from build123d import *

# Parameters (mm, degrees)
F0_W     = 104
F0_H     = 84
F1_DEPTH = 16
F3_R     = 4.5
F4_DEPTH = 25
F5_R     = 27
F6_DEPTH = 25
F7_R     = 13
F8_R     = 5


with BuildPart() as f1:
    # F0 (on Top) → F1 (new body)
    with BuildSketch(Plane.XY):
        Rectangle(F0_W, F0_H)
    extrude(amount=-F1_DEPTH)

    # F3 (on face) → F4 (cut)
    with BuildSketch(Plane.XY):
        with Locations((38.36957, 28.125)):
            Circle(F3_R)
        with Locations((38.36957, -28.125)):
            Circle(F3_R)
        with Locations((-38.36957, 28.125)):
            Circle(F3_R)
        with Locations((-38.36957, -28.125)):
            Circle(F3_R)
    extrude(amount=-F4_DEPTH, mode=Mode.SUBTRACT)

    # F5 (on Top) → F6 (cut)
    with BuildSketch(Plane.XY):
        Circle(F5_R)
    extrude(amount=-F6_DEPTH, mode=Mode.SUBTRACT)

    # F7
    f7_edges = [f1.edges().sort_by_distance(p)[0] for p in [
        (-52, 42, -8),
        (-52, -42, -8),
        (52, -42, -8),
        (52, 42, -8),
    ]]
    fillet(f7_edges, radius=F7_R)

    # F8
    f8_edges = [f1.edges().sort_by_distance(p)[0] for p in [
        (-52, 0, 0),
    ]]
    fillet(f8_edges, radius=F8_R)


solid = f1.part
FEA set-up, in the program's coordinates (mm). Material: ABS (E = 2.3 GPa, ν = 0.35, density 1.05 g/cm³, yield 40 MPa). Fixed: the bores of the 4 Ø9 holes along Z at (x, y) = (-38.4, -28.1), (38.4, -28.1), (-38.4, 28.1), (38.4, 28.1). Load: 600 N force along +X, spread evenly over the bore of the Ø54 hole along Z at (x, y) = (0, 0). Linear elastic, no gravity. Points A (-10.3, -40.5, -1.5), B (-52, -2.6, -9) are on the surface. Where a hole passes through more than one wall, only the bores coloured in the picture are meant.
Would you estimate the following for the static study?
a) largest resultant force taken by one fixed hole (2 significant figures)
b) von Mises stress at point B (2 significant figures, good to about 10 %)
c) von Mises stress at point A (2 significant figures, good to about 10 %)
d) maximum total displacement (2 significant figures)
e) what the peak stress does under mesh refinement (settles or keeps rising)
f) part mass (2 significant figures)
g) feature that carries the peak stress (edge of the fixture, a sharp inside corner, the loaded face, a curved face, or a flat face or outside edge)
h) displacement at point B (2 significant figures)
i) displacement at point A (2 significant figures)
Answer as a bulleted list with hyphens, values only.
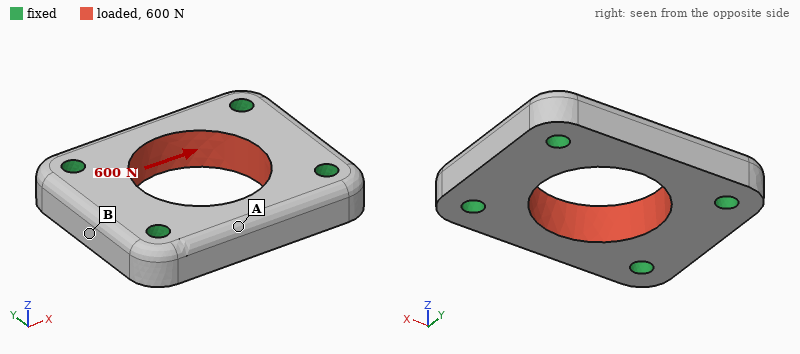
- 150 N
- 0.33 MPa
- 0.12 MPa
- 6.2 µm
- keeps rising
- 100 g
- edge of the fixture
- 4.7 µm
- 2.2 µm
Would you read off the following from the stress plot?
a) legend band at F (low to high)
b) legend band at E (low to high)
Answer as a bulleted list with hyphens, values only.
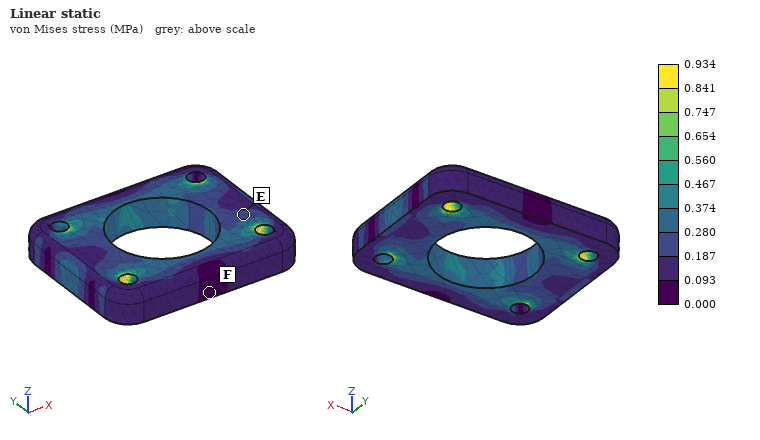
- 0.000 to 0.093 MPa
- 0.187 to 0.280 MPa
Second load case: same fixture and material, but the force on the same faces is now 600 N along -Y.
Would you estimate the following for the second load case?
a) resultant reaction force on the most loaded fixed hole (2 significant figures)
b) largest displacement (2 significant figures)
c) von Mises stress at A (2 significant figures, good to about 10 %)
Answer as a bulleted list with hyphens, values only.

- 150 N
- 16 µm
- 0.48 MPa
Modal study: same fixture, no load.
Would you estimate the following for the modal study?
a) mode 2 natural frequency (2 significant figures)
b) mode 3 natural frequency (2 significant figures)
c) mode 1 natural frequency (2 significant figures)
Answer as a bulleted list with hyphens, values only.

- 3900 Hz
- 4300 Hz
- 3800 Hz
